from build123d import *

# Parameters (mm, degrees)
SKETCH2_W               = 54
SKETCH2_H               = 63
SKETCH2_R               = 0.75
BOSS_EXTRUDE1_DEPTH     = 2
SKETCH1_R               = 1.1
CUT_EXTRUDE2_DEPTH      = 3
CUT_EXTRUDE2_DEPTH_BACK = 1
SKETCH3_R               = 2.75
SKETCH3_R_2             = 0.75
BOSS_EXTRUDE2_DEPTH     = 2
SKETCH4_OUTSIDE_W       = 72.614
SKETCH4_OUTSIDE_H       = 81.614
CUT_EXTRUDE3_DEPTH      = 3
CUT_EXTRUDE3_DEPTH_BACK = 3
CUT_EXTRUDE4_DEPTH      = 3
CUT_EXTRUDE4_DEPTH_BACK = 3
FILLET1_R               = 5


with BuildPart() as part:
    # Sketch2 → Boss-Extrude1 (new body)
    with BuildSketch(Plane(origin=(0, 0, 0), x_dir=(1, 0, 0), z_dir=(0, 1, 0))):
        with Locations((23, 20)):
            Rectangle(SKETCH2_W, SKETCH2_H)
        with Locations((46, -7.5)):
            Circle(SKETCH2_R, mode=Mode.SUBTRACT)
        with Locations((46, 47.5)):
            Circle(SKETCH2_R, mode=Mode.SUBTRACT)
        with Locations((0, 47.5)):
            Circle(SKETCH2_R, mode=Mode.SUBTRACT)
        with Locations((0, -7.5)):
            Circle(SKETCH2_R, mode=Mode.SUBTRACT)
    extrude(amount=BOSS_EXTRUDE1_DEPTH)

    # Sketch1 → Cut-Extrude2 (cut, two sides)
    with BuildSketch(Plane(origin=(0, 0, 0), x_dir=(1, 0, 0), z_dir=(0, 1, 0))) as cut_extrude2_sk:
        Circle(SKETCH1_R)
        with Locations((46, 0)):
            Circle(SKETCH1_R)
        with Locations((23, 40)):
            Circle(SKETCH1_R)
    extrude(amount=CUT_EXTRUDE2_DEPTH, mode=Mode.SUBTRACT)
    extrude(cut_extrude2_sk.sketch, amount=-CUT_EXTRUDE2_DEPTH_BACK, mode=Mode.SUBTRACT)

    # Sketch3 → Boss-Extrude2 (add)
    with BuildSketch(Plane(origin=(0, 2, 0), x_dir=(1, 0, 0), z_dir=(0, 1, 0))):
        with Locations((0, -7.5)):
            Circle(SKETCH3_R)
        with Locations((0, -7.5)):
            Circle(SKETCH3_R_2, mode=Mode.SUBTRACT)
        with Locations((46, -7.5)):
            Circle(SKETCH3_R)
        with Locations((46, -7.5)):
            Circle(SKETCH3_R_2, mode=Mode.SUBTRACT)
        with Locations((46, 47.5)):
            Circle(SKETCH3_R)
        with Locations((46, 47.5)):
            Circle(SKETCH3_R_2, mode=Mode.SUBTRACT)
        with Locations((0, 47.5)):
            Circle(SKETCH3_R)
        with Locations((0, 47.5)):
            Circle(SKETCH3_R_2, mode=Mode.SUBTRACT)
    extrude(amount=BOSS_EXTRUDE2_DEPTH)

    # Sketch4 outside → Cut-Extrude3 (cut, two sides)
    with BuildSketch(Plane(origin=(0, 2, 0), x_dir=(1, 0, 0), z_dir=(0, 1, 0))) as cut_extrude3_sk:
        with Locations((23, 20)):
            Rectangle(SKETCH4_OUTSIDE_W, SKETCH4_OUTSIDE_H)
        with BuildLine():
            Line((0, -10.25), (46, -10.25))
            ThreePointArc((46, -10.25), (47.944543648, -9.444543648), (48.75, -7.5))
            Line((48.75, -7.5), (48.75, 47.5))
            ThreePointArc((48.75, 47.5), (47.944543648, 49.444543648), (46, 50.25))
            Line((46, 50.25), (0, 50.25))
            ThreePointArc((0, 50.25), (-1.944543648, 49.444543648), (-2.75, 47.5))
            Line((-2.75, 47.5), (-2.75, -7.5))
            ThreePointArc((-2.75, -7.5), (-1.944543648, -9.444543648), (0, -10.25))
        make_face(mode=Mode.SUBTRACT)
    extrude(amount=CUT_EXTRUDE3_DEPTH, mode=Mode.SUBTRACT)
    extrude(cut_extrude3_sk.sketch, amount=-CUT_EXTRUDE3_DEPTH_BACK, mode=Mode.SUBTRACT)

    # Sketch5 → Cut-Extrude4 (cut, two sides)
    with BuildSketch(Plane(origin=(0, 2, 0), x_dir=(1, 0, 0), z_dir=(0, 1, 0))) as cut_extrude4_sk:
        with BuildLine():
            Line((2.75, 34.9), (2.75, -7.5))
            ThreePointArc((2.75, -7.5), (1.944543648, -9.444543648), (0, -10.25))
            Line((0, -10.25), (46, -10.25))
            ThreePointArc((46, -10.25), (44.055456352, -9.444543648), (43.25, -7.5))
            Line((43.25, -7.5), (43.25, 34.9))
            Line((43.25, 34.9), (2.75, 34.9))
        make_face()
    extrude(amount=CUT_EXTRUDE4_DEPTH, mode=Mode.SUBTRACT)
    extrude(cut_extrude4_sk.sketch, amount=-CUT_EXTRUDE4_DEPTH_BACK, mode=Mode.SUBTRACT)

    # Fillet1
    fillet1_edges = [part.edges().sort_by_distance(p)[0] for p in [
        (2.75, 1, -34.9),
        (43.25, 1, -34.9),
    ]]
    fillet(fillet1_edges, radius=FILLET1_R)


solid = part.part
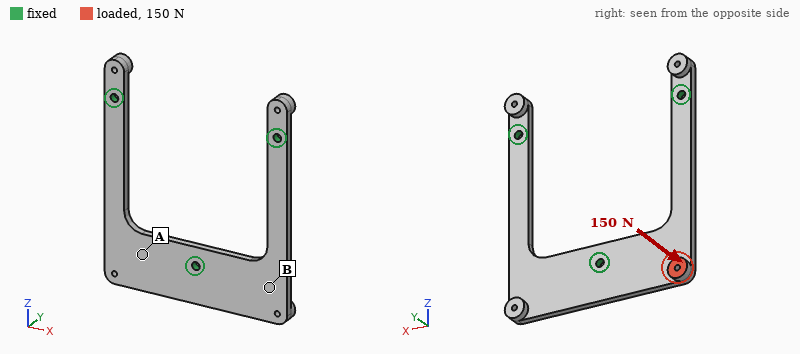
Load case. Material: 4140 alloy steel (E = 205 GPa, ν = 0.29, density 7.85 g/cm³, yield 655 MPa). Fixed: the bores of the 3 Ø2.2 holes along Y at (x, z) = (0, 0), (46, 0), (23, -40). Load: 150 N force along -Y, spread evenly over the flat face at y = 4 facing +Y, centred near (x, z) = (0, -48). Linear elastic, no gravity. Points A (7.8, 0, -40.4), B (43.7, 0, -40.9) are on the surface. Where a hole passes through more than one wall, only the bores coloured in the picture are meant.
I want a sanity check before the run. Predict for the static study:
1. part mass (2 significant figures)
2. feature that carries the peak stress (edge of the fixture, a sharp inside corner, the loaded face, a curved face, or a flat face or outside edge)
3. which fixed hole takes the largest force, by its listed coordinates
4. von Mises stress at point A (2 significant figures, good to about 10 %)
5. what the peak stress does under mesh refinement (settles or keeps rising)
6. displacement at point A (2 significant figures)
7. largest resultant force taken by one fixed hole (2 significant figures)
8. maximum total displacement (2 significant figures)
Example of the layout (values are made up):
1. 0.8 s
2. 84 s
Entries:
1. 21 g
2. edge of the fixture
3. (23, -40)
4. 98 MPa
5. keeps rising
6. 0.13 mm
7. 140 N
8. 0.35 mm
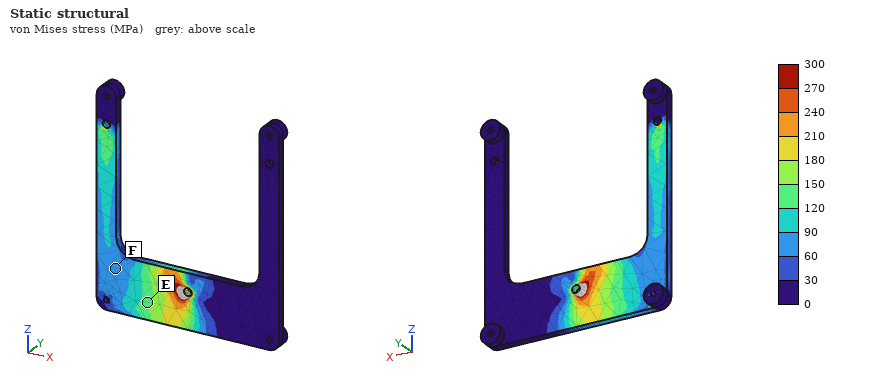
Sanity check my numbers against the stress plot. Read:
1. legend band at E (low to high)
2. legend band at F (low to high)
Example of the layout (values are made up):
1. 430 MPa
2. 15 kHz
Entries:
1. 120 to 150 MPa
2. 60 to 90 MPa
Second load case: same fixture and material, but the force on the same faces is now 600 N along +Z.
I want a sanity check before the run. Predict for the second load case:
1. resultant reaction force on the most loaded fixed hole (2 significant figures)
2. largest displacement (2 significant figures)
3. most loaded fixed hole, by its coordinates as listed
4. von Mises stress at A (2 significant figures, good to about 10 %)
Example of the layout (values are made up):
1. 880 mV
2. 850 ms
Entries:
1. 490 N
2. 0.14 mm
3. (0, 0)
4. 82 MPa
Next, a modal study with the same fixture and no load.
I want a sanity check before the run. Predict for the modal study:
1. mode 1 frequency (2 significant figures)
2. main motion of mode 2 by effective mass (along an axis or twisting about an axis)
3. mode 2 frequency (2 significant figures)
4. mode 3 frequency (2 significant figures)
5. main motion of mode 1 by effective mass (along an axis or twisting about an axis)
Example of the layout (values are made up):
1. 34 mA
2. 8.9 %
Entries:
1. 2100 Hz
2. along Y
3. 2400 Hz
4. 5100 Hz
5. twisting about Z
